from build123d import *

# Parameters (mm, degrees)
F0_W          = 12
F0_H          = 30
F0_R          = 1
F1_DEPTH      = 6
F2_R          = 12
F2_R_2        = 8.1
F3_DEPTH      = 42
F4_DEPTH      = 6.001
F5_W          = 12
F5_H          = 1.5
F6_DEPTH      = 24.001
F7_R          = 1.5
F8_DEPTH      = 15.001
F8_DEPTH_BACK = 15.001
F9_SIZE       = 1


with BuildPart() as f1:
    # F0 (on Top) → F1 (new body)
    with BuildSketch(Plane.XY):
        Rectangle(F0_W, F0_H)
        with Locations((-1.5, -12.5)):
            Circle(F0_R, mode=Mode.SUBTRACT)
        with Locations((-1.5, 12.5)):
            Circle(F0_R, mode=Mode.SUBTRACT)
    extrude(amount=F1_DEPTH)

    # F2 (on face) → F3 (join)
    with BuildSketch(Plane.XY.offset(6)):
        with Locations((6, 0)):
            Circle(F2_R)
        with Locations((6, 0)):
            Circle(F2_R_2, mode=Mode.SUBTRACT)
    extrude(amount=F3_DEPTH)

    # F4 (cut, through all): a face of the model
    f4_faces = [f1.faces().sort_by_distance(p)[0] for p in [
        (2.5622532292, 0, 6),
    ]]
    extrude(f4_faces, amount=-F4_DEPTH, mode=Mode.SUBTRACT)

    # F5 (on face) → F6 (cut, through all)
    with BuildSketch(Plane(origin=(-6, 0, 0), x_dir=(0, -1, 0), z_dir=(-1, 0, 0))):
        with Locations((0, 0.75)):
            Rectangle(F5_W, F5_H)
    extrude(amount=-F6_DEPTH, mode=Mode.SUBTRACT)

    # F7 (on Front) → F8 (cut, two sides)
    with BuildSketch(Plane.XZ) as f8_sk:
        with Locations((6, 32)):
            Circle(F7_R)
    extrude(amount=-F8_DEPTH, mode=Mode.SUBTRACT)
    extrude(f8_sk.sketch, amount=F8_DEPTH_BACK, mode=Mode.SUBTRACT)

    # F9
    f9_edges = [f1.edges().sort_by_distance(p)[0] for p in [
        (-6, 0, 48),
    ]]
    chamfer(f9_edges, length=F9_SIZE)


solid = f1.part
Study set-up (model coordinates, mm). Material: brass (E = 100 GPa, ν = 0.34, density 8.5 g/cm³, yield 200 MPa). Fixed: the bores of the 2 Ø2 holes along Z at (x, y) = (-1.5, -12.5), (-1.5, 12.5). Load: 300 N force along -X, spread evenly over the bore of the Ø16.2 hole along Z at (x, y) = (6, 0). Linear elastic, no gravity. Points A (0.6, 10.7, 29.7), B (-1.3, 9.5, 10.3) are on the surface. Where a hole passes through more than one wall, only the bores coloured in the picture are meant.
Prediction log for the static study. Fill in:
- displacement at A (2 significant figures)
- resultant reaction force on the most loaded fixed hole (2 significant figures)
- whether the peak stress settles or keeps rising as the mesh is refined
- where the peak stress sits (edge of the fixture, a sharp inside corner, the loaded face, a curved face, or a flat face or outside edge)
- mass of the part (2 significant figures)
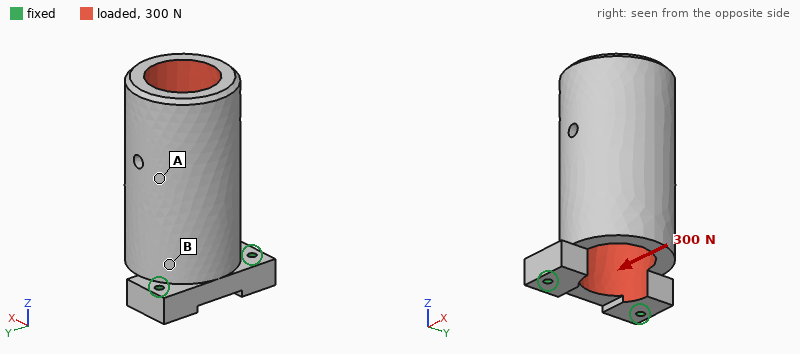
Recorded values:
38 µm
150 N
keeps rising
edge of the fixture
99 g
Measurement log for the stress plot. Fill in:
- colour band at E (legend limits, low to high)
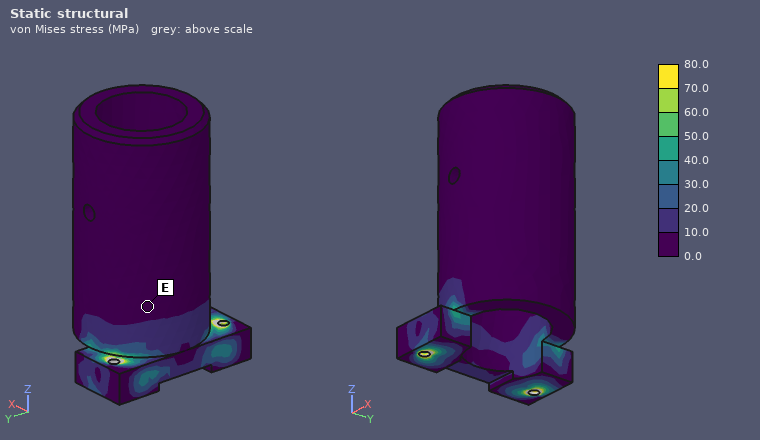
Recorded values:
0.0 to 10.0 MPa
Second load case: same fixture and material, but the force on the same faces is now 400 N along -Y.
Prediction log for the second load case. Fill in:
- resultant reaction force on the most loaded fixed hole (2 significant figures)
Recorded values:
450 N
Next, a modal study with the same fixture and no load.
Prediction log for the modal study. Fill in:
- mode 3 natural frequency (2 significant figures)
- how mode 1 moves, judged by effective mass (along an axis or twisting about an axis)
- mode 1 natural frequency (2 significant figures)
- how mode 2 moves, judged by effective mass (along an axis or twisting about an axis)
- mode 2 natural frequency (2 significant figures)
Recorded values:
6200 Hz
along X
1300 Hz
along Y
3500 Hz
